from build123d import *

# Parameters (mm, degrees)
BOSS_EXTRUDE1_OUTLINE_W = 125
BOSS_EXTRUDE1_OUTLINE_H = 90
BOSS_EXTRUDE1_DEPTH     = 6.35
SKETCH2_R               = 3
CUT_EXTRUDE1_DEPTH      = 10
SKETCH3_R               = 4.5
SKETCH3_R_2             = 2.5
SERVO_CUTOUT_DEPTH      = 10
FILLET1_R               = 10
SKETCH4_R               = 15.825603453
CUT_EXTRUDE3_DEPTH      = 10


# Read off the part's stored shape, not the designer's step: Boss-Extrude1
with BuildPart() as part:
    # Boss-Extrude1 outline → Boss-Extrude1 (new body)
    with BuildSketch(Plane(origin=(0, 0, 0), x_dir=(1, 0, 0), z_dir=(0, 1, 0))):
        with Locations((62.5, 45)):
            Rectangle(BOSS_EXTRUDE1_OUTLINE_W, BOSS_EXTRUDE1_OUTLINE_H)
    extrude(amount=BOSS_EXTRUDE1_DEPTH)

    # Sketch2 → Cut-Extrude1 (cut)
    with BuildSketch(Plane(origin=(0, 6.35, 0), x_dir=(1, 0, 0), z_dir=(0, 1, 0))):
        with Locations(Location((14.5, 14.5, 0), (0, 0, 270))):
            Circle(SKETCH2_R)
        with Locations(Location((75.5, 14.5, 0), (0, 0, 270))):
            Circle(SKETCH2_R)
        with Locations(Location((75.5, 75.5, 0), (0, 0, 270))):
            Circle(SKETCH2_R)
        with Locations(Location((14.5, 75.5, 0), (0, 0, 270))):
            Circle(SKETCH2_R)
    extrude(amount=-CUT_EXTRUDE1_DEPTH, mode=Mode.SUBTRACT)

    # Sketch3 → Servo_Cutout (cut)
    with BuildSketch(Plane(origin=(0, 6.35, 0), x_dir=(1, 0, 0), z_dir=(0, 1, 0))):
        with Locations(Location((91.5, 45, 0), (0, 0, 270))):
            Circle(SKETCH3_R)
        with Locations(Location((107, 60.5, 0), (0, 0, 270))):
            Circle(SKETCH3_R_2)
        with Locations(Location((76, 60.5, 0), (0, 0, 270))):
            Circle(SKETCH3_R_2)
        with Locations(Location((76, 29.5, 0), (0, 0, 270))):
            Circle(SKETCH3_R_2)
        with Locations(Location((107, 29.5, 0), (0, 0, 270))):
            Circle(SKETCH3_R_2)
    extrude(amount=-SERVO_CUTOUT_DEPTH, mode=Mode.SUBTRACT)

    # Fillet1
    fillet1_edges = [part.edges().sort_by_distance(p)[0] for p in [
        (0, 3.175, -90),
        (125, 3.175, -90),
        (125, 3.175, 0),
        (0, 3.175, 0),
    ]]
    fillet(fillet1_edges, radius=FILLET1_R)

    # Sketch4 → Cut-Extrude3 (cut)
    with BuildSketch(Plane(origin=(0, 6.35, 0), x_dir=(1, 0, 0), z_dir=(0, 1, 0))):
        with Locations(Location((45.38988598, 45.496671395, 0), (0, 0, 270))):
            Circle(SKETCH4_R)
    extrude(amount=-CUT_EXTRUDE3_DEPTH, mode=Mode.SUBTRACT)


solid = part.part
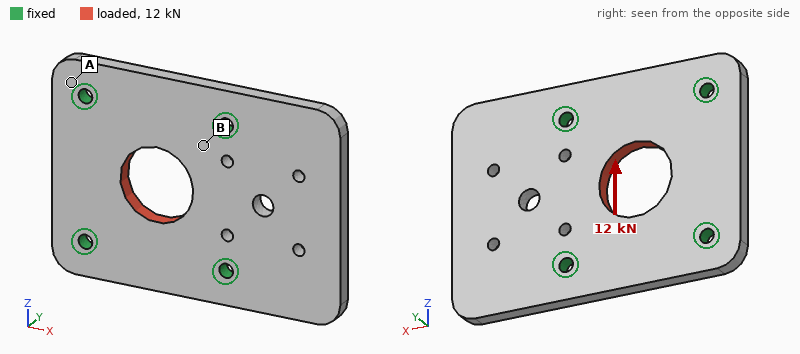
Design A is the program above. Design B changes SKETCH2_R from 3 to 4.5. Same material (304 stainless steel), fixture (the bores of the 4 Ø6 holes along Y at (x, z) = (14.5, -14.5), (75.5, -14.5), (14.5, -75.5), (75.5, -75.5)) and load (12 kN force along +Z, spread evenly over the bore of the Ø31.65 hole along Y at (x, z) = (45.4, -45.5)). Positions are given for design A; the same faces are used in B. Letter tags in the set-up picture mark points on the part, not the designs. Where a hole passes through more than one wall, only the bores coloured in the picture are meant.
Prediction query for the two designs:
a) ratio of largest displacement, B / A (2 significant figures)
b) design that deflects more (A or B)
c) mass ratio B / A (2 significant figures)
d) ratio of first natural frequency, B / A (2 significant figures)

0.91
A
0.99
1.1
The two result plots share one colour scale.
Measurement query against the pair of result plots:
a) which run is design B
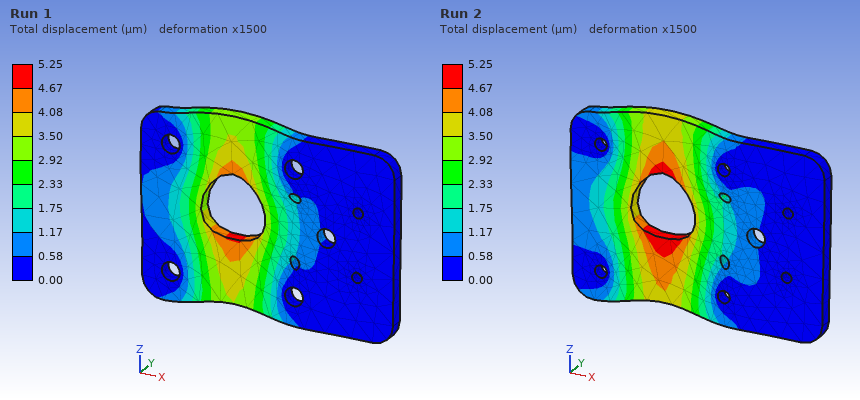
Run 1
